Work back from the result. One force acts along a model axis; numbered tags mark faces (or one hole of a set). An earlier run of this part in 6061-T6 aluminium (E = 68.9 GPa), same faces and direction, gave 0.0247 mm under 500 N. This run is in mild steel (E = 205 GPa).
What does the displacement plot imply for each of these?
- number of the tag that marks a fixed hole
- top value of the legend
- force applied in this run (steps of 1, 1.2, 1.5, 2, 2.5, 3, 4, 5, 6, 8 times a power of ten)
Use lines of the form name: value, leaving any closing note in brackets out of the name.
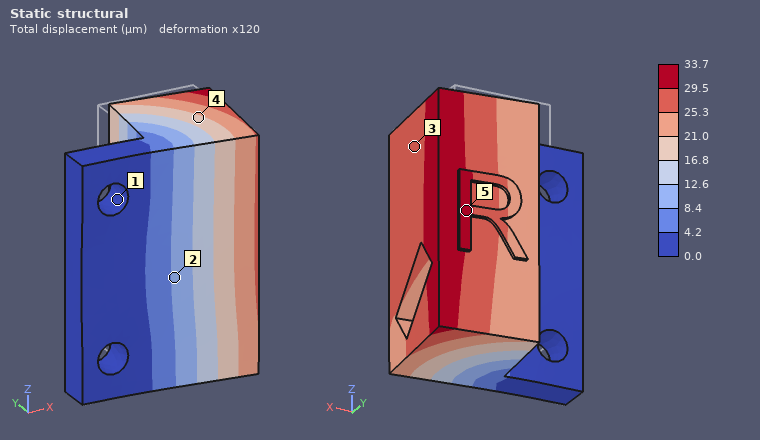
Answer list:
number of the tag that marks a fixed hole: 1
top value of the legend: 33.7 µm
force applied in this run: 2 kN
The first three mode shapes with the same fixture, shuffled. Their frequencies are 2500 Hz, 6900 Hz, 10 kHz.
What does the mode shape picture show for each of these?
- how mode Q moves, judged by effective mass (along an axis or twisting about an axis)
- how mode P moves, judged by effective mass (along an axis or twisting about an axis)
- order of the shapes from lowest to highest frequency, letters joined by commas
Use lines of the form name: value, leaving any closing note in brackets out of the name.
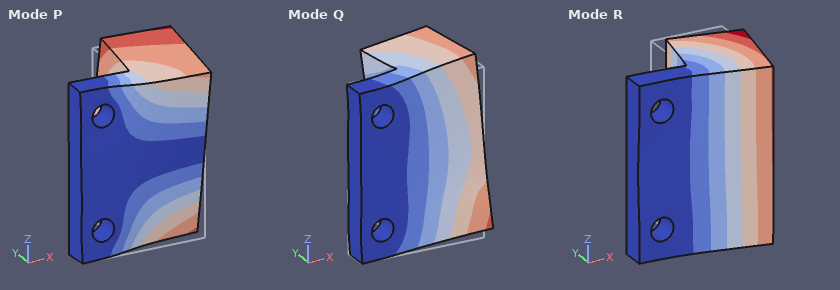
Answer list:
how mode Q moves, judged by effective mass: along Z
how mode P moves, judged by effective mass: along Z
order of the shapes from lowest to highest frequency, letters joined by commas: R, P, Q
